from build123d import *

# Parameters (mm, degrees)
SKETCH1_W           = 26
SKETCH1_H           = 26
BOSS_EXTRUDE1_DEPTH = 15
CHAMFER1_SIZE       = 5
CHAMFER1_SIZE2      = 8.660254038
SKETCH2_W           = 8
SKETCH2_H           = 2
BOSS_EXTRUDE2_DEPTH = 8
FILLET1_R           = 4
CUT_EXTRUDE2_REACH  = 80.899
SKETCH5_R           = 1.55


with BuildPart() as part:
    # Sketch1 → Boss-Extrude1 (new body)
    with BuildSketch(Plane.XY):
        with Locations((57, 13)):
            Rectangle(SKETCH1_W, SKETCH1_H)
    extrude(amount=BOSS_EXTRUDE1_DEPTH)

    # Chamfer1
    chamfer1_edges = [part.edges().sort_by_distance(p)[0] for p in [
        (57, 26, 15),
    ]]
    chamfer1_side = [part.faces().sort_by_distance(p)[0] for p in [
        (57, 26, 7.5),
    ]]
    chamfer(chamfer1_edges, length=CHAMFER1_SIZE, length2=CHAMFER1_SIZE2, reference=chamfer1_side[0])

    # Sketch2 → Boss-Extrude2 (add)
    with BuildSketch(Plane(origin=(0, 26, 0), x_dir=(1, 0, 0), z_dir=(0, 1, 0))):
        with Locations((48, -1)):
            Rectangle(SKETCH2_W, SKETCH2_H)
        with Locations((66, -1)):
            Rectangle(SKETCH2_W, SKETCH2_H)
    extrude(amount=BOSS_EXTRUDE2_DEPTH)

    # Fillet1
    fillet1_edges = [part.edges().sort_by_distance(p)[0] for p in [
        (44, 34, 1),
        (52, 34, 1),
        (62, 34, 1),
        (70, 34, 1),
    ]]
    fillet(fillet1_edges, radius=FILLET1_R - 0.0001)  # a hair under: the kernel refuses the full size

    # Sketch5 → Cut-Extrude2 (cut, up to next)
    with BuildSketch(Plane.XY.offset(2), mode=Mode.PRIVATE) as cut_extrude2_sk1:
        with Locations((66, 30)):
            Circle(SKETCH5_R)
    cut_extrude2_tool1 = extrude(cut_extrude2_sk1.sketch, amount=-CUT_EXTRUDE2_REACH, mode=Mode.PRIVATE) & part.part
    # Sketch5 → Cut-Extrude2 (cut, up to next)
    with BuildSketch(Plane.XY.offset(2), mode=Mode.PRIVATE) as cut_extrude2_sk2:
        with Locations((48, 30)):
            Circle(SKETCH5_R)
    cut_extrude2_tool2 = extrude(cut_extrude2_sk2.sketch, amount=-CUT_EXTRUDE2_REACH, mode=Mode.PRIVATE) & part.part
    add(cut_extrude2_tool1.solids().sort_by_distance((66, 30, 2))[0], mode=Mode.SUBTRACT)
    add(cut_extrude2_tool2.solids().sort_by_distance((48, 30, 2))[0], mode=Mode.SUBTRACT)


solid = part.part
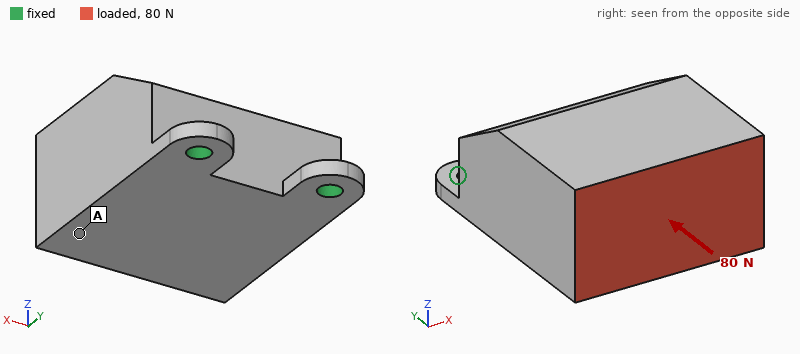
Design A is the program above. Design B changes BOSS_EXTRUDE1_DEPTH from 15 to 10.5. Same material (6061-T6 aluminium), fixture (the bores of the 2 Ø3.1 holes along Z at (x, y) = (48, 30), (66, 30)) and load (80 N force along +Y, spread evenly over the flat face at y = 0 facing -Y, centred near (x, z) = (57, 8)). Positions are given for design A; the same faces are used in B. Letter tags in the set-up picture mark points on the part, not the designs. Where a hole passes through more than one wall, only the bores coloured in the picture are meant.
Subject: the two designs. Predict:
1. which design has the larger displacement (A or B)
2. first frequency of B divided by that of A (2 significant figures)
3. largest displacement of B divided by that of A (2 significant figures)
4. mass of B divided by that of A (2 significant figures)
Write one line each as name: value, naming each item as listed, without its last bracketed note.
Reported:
which design has the larger displacement: A
first frequency of B divided by that of A: 1.3
largest displacement of B divided by that of A: 0.61
mass of B divided by that of A: 0.69
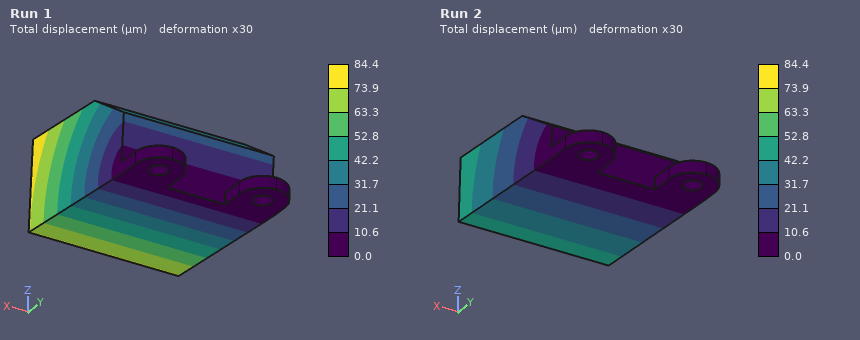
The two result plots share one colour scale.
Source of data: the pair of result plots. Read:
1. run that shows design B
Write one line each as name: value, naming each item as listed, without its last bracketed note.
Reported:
run that shows design B: Run 2
